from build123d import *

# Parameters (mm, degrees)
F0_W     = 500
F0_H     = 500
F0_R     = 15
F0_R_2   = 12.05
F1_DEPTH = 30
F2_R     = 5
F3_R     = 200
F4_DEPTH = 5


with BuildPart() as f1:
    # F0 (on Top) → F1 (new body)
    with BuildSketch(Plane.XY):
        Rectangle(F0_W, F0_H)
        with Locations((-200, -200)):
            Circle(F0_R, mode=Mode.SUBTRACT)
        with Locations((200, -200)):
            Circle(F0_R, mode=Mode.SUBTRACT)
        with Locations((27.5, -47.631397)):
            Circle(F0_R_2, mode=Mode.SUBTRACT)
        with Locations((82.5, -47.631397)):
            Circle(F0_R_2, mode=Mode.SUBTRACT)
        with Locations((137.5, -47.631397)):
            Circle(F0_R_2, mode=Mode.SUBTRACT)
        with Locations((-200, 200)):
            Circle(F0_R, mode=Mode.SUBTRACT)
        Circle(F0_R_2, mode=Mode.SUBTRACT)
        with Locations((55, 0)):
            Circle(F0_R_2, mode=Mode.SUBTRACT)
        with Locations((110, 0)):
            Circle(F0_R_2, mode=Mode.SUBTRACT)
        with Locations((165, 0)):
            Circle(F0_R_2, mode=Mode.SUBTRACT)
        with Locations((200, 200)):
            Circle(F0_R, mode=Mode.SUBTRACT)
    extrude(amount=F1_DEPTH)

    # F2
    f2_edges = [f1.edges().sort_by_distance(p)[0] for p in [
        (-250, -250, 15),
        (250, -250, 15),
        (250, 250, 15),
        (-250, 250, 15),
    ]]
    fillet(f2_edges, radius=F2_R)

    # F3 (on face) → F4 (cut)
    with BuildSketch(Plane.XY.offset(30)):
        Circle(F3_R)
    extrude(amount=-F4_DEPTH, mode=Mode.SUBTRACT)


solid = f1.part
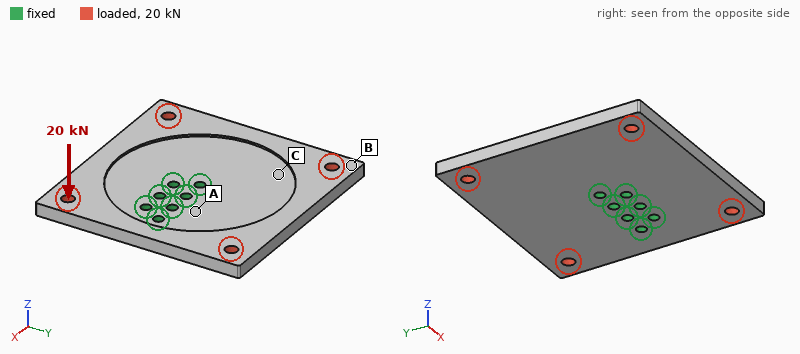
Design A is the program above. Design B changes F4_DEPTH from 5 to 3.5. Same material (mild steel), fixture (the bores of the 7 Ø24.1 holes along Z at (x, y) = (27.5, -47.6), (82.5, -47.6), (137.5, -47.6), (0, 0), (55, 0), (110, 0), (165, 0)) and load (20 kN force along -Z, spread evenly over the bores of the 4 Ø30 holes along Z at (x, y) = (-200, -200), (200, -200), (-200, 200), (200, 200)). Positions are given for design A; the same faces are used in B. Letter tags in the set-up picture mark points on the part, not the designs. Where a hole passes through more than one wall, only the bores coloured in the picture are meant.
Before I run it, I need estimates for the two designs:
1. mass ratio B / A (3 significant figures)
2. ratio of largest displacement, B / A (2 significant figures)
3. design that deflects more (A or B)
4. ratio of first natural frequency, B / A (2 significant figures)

1.03
0.88
A
1.1
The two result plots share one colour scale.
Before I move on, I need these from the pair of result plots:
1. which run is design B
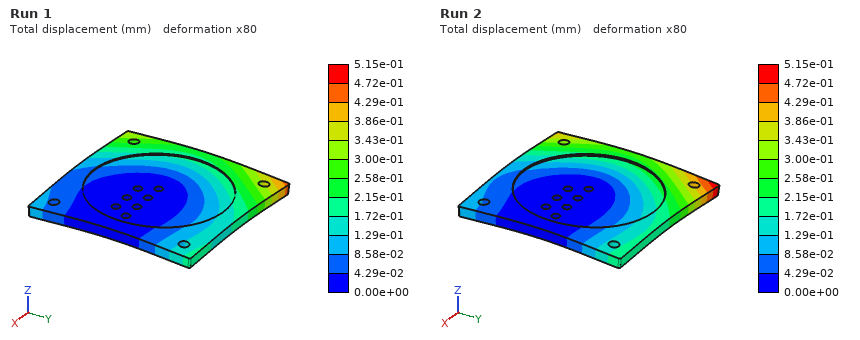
Run 1
